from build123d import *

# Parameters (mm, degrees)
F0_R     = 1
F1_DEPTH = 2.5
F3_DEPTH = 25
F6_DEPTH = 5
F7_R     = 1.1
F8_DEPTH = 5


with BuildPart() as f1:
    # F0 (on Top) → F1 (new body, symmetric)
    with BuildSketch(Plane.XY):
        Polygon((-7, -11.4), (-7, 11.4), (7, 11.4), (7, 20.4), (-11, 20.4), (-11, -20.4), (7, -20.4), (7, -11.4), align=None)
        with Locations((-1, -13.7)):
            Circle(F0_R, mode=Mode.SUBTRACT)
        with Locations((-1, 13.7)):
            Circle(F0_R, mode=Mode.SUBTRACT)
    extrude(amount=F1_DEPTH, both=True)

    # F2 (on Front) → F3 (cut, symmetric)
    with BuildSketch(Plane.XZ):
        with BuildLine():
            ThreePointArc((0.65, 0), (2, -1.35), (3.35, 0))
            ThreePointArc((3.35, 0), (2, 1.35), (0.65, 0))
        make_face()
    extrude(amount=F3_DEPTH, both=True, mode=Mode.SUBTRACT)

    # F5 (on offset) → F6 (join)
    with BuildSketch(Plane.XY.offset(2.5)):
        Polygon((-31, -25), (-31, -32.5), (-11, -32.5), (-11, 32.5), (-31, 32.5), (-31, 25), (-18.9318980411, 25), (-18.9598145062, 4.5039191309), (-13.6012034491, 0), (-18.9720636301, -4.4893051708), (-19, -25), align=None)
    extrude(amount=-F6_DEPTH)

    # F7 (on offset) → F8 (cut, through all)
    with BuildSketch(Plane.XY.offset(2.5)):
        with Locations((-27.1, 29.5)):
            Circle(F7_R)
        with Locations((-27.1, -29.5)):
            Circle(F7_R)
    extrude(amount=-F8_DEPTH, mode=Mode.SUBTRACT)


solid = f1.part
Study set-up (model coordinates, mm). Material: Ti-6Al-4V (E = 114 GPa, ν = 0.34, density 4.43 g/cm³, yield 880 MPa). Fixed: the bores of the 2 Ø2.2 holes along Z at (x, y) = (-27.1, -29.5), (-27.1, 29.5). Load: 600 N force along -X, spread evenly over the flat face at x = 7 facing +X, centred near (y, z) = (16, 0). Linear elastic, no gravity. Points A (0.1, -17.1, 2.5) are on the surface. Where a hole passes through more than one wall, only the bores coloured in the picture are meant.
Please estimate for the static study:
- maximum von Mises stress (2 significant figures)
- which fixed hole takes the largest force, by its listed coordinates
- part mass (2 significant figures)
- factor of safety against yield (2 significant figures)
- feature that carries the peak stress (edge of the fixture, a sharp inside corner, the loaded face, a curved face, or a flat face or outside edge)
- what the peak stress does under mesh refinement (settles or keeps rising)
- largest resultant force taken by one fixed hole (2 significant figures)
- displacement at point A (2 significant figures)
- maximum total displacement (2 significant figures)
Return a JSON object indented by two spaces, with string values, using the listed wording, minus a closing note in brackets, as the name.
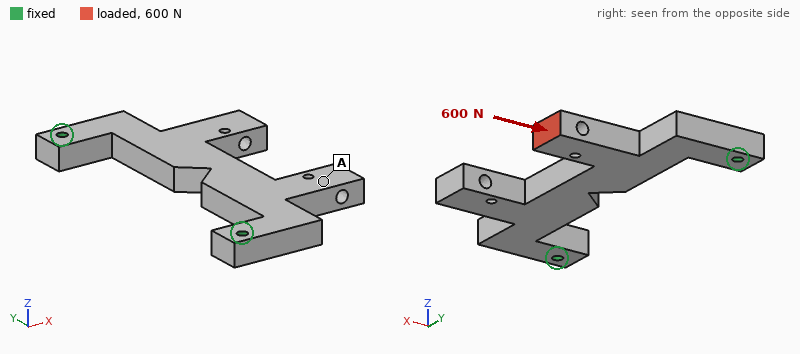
{
  "maximum von Mises stress": "62 MPa",
  "which fixed hole takes the largest force, by its listed coordinates": "(-27.1, 29.5)",
  "part mass": "23 g",
  "factor of safety against yield": "14",
  "feature that carries the peak stress": "a curved face",
  "what the peak stress does under mesh refinement": "settles",
  "largest resultant force taken by one fixed hole": "530 N",
  "displacement at point A": "3.9 µm",
  "maximum total displacement": "16 µm"
}
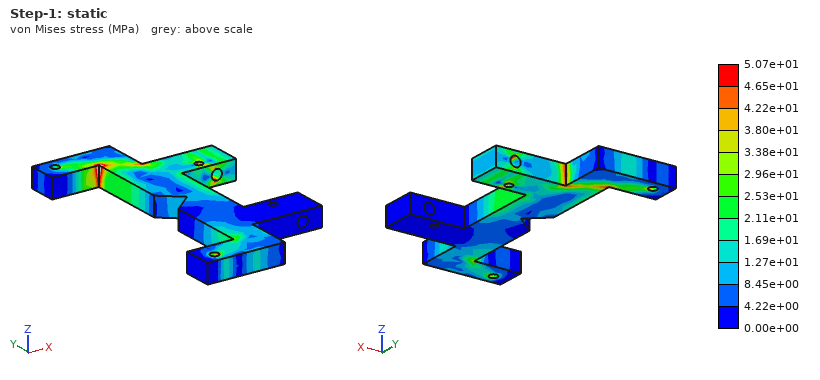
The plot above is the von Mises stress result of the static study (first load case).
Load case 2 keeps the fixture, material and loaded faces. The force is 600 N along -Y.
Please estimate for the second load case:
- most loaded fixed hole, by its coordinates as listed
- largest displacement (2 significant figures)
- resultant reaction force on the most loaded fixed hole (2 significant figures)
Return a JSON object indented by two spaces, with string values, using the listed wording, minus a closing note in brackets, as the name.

{
  "most loaded fixed hole, by its coordinates as listed": "(-27.1, -29.5)",
  "largest displacement": "77 µm",
  "resultant reaction force on the most loaded fixed hole": "590 N"
}
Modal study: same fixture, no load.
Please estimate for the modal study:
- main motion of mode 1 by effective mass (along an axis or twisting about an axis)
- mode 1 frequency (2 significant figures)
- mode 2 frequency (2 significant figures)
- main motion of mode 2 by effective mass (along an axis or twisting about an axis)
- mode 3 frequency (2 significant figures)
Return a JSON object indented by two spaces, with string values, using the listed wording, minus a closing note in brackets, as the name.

{
  "main motion of mode 1 by effective mass": "along Z",
  "mode 1 frequency": "2500 Hz",
  "mode 2 frequency": "5200 Hz",
  "main motion of mode 2 by effective mass": "twisting about X",
  "mode 3 frequency": "6700 Hz"
}
